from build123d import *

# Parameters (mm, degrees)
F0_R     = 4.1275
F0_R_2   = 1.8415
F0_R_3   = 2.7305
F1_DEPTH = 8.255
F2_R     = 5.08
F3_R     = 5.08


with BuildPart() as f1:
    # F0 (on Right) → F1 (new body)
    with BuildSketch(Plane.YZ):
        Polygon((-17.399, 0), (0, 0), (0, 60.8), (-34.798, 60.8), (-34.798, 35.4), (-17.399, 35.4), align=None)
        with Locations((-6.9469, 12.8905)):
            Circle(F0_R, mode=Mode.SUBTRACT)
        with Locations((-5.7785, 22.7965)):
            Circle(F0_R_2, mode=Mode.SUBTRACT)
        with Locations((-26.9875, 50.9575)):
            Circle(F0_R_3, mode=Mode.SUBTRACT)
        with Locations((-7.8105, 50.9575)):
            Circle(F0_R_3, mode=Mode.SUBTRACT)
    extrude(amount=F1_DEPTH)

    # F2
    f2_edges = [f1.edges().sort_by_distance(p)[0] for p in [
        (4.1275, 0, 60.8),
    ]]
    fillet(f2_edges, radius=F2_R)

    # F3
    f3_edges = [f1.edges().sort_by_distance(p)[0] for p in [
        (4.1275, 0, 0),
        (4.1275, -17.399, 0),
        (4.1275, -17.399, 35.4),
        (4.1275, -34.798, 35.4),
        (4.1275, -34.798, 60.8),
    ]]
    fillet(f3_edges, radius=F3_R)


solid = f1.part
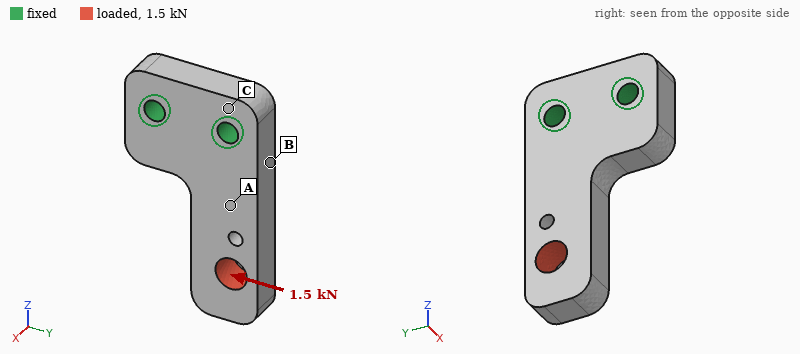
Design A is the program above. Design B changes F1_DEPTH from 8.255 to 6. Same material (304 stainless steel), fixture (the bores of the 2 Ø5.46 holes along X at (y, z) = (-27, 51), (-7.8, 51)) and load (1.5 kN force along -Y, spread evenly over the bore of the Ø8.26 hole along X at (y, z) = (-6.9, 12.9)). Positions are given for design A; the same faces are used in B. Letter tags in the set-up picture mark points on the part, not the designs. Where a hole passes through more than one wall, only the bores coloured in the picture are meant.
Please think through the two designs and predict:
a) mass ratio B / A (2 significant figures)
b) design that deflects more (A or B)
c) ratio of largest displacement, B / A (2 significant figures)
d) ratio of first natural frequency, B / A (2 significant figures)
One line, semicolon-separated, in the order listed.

0.73; B; 1.4; 0.75
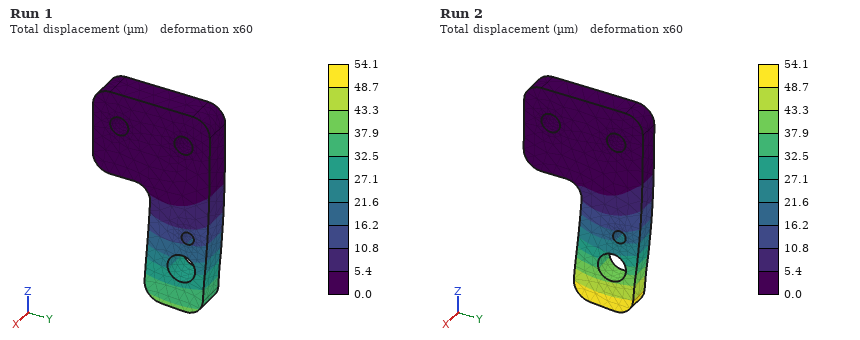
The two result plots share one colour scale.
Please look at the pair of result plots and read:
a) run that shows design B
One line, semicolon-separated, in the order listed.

Run 2
